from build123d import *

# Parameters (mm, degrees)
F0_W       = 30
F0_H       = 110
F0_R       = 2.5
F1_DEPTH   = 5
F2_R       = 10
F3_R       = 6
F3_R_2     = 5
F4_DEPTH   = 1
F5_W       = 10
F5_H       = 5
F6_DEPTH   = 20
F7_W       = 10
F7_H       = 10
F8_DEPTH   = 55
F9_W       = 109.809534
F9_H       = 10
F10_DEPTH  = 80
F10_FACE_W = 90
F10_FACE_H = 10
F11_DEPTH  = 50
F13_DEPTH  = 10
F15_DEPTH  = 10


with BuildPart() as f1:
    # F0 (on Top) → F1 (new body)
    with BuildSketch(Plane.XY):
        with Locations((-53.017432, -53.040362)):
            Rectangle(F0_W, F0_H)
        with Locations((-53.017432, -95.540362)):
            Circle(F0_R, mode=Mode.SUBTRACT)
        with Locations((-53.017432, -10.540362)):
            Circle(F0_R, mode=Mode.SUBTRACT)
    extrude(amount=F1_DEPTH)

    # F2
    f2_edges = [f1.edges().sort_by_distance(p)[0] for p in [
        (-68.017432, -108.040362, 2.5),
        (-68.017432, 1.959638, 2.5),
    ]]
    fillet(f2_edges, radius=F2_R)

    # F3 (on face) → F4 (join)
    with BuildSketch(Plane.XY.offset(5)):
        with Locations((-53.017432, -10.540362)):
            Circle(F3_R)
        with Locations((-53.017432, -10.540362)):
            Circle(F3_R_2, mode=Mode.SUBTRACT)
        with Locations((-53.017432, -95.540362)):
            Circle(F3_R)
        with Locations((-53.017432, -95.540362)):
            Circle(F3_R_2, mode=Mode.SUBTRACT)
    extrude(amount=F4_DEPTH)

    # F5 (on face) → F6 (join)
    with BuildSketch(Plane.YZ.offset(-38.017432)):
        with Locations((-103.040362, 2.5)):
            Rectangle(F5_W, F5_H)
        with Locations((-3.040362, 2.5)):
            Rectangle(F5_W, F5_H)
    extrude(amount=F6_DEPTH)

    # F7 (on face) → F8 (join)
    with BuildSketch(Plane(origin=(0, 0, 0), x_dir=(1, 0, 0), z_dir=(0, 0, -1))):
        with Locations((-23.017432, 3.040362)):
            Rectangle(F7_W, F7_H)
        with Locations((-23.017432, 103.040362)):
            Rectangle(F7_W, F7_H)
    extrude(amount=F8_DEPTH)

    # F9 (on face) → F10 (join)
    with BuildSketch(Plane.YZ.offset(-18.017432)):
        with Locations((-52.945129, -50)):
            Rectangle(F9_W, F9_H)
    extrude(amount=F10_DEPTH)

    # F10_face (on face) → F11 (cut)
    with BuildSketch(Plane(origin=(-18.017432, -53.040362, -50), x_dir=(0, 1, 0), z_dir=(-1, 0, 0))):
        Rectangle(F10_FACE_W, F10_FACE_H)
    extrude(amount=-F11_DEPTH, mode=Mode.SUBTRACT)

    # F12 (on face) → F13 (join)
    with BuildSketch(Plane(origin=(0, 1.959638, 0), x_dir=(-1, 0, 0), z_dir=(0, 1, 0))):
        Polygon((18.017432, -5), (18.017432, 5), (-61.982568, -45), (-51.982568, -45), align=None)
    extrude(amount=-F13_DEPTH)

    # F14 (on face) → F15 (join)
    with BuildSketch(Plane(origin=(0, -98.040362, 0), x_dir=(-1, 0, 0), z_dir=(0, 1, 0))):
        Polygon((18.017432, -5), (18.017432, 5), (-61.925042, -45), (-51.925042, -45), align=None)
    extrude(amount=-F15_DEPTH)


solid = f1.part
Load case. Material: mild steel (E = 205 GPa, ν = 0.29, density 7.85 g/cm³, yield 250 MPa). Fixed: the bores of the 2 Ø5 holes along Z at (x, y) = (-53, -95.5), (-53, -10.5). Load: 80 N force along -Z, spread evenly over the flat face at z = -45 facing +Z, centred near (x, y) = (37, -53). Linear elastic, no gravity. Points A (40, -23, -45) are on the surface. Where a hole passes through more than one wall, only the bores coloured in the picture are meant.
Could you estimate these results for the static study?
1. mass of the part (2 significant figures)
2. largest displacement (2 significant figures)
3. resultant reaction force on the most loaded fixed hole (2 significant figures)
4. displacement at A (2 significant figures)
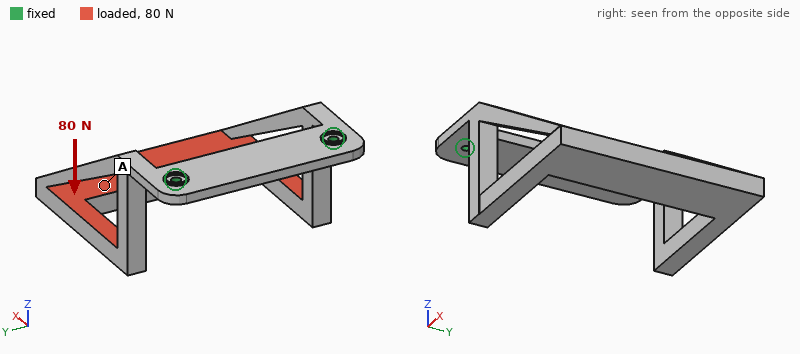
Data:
660 g
0.36 mm
40 N
0.28 mm
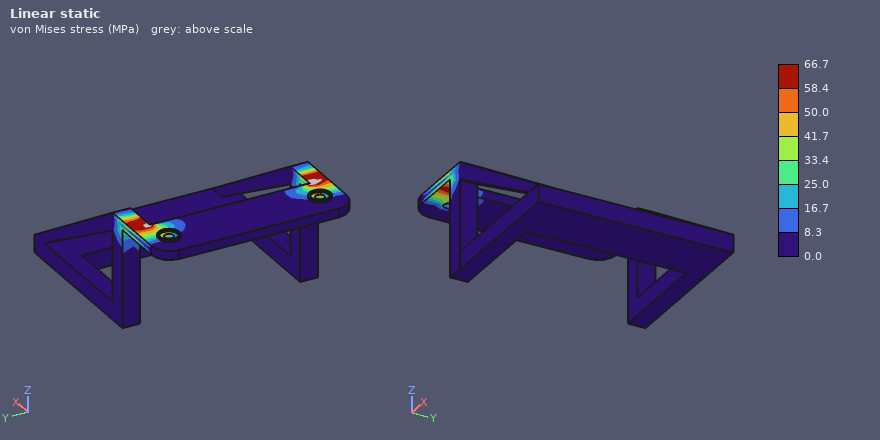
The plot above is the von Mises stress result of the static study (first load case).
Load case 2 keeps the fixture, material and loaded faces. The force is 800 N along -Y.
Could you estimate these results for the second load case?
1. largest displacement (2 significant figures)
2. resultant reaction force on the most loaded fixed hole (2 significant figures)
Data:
0.40 mm
900 N
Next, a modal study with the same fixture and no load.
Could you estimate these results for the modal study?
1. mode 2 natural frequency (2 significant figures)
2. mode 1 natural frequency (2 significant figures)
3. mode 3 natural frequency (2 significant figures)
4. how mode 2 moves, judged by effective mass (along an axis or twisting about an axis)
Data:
350 Hz
120 Hz
550 Hz
along Y
